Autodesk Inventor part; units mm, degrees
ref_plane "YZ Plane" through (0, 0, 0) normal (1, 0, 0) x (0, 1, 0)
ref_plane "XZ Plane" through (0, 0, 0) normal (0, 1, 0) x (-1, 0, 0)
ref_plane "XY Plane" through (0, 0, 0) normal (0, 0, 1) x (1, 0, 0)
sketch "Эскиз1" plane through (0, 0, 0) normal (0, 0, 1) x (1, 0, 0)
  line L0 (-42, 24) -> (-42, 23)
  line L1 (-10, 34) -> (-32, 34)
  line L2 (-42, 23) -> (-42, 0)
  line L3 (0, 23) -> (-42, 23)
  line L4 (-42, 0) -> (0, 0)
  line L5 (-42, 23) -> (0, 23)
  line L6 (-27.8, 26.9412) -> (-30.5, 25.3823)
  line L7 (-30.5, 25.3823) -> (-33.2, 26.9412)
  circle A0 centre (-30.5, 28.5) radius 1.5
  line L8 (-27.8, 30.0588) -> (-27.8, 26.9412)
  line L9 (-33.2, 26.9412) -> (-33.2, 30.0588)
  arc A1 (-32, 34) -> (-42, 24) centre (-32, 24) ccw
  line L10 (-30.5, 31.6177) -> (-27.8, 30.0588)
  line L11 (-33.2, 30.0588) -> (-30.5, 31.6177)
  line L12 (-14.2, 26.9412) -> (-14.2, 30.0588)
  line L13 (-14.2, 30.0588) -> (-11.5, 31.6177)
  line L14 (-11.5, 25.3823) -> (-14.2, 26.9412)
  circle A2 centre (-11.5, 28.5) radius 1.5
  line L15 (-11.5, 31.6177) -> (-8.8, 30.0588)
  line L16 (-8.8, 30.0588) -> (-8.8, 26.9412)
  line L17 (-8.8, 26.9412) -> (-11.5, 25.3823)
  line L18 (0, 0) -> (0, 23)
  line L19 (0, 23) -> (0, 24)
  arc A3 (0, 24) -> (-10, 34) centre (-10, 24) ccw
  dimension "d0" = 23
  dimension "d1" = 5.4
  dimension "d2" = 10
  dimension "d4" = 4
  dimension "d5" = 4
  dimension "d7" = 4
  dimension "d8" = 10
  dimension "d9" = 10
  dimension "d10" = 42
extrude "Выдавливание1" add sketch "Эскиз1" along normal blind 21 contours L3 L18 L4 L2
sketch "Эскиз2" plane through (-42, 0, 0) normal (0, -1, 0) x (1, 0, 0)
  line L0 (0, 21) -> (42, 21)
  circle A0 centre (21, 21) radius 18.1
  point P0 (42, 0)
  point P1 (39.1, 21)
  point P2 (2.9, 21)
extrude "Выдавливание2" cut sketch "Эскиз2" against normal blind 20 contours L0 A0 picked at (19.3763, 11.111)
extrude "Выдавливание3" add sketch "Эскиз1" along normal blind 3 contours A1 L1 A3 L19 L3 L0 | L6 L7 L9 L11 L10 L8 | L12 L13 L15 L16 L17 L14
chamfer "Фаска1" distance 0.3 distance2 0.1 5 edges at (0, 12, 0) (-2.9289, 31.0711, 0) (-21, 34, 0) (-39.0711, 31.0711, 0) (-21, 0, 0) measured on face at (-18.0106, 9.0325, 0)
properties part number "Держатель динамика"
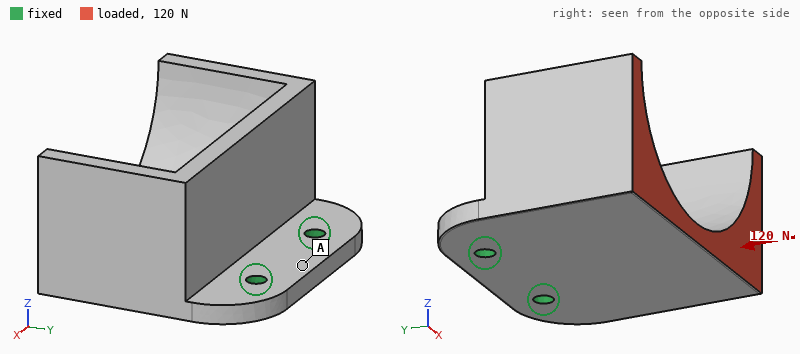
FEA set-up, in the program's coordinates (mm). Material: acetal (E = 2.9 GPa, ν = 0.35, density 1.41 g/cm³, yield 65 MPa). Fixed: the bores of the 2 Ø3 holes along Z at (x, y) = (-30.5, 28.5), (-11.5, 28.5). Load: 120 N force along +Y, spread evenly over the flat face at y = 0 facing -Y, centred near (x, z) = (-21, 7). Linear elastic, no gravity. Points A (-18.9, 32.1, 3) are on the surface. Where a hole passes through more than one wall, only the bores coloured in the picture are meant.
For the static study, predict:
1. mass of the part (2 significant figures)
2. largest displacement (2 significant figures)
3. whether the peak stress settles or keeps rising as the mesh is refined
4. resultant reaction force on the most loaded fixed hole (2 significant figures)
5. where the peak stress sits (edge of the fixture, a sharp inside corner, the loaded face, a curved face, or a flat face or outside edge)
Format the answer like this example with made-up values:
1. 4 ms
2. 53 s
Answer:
1. 16 g
2. 0.59 mm
3. keeps rising
4. 60 N
5. edge of the fixture
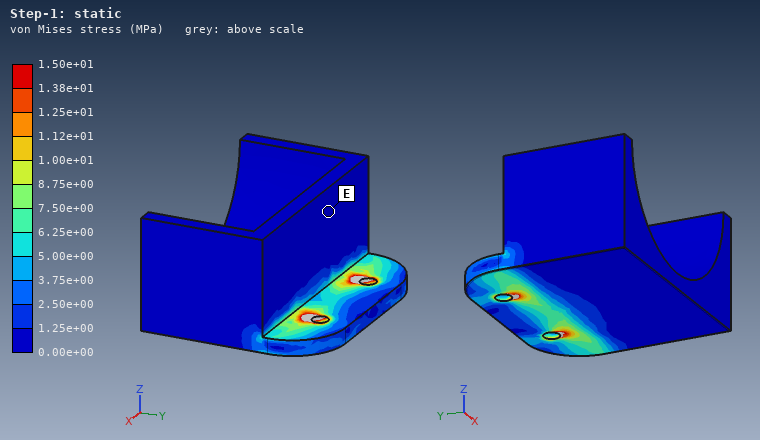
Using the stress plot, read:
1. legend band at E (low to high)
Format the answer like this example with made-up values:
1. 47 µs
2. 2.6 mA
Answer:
1. 0.00e+00 to 1.25e+00 MPa
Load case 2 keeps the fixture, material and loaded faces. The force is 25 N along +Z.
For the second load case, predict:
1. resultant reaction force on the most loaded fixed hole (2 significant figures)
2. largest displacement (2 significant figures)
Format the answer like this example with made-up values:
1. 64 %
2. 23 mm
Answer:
1. 13 N
2. 0.61 mm
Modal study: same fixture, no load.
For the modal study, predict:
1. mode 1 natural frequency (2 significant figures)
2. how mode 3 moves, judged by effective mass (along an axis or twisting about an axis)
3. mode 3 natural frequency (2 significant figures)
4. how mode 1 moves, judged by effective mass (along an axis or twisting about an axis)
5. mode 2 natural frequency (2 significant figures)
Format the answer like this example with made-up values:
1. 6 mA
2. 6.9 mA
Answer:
1. 470 Hz
2. along X
3. 2100 Hz
4. along Z
5. 1100 Hz
